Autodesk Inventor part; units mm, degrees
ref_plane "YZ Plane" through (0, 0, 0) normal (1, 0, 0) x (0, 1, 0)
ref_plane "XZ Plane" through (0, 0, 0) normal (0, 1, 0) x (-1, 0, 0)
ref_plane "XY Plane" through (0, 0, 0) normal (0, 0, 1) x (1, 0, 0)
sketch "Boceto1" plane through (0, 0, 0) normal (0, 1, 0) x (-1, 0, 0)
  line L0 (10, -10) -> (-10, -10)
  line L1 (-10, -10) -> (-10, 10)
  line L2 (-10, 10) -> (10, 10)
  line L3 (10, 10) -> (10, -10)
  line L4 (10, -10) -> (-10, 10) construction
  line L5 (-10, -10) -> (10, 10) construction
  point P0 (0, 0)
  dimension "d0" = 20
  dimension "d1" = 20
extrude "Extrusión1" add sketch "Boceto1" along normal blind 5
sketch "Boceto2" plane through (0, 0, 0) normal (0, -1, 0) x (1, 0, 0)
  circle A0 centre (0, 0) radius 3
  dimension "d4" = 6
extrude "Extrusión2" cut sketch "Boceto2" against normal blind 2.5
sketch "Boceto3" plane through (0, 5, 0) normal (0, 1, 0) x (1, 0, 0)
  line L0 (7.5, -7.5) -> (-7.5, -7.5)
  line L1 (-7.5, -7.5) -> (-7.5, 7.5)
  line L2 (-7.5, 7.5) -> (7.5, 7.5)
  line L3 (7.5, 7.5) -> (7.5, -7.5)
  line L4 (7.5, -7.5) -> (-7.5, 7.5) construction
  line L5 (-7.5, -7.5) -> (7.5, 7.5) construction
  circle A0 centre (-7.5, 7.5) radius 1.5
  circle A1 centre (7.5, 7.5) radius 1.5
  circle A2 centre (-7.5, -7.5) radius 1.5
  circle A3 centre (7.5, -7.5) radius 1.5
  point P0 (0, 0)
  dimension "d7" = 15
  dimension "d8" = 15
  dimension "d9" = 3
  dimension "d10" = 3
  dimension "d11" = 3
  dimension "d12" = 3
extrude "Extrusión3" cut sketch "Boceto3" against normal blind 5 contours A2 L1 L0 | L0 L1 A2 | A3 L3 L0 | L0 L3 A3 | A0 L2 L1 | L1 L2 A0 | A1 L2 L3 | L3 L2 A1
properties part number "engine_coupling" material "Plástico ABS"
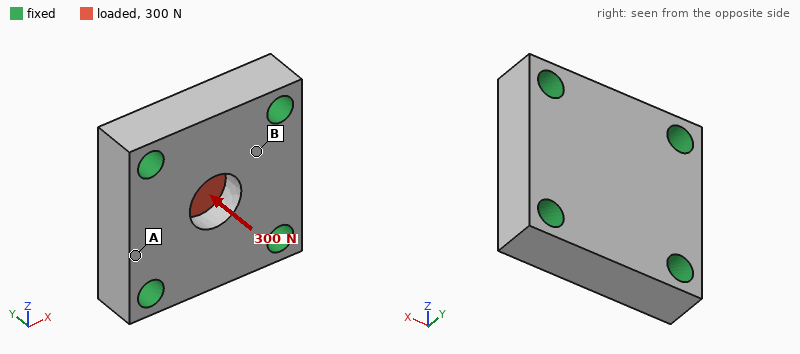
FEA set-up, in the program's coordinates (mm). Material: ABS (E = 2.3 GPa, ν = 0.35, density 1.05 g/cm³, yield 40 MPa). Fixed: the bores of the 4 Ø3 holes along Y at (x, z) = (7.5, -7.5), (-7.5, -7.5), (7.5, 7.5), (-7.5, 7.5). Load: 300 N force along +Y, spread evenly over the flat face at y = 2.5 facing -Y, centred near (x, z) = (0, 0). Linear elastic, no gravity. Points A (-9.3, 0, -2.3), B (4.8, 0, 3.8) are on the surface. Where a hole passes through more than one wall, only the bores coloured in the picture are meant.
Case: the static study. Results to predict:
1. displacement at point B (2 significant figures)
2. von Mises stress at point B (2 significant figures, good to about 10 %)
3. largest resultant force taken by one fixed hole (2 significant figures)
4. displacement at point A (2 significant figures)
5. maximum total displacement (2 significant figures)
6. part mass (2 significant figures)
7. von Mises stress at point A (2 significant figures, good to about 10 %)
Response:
24 µm
5.9 MPa
77 N
12 µm
77 µm
1.9 g
2.3 MPa
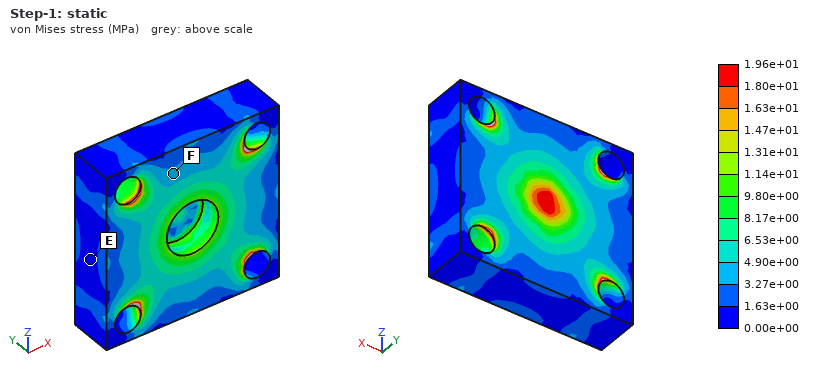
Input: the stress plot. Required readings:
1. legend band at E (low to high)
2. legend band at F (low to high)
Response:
0.00e+00 to 1.63e+00 MPa
3.27e+00 to 4.90e+00 MPa
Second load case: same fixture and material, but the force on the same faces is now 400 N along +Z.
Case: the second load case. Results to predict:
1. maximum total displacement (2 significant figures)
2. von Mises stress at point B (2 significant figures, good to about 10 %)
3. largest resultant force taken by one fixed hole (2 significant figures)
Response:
46 µm
3.2 MPa
110 N
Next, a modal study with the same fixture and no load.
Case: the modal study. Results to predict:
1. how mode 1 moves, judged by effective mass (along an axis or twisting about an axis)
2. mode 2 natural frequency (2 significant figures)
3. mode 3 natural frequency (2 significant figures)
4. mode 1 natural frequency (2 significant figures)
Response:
along Y
27 kHz
27 kHz
19 kHz
